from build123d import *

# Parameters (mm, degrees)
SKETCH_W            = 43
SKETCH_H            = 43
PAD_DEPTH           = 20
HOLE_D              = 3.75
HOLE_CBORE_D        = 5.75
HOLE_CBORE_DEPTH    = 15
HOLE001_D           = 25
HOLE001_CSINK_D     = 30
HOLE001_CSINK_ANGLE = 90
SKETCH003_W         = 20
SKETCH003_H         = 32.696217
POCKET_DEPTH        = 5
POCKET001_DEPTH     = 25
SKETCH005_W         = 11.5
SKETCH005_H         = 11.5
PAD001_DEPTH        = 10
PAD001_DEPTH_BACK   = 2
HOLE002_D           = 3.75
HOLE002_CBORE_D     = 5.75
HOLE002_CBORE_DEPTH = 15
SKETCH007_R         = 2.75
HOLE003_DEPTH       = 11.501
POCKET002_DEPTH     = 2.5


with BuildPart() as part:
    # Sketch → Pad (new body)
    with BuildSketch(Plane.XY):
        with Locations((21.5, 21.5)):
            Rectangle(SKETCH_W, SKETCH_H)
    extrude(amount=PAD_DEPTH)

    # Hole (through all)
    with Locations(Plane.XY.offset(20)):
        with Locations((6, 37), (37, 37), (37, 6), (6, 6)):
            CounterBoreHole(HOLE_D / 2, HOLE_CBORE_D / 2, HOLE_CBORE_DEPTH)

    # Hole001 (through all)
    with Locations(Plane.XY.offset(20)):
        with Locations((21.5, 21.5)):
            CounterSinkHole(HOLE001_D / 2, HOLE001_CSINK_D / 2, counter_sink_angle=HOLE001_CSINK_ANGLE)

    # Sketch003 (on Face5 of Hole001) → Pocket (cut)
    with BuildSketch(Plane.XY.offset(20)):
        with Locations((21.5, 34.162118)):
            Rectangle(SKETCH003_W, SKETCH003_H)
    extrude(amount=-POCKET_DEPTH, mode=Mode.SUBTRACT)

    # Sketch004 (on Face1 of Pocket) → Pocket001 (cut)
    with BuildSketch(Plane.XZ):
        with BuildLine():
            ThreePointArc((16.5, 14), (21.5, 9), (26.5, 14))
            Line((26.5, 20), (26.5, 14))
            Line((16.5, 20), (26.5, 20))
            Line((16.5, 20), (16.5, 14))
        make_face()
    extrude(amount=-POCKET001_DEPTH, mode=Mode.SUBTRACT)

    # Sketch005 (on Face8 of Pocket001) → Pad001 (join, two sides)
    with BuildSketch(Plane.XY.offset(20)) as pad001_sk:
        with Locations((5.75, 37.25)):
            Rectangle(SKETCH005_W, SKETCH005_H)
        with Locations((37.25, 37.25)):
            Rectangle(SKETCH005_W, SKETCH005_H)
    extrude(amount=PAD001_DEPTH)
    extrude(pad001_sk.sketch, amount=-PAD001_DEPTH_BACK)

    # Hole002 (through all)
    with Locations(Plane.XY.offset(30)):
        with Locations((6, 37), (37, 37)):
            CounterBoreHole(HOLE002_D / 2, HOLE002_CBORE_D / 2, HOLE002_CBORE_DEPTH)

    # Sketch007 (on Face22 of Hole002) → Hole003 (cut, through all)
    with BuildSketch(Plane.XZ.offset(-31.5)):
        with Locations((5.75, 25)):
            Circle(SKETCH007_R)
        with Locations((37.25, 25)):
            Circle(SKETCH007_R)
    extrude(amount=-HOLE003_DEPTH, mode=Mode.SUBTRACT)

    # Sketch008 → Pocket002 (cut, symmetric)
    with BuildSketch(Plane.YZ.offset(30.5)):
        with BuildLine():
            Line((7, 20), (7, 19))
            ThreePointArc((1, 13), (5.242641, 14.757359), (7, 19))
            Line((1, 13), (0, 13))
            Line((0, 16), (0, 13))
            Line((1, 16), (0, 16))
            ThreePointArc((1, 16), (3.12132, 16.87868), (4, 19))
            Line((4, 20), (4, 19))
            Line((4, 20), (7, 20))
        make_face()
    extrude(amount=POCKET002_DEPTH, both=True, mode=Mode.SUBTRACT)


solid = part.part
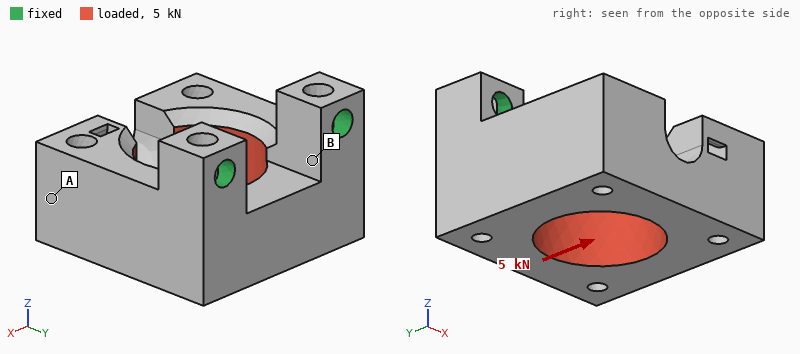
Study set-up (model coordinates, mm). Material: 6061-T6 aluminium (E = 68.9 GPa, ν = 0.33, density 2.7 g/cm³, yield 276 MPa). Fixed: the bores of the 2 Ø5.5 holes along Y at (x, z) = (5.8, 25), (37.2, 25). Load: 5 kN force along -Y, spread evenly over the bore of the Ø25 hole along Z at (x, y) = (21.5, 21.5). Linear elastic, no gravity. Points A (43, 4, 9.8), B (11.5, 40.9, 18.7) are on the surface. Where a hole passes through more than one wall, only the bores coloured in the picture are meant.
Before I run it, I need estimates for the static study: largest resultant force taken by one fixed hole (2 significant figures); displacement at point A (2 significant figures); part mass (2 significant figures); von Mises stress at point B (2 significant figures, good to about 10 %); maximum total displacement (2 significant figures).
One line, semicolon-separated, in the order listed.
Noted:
2.5 kN; 0.12 mm; 67 g; 68 MPa; 0.15 mm
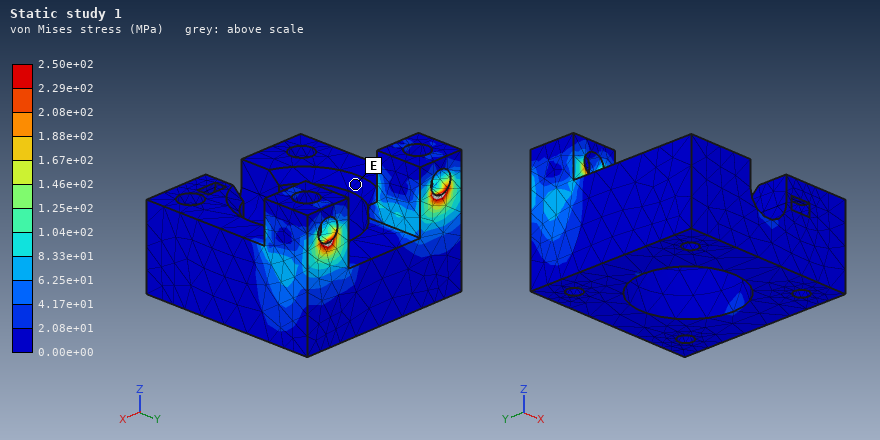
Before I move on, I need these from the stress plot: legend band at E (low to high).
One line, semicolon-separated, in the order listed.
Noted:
0.00e+00 to 2.08e+01 MPa
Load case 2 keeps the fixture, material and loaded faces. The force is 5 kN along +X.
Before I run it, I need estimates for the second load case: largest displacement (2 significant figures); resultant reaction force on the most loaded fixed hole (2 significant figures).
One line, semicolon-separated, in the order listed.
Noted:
86 µm; 3.4 kN
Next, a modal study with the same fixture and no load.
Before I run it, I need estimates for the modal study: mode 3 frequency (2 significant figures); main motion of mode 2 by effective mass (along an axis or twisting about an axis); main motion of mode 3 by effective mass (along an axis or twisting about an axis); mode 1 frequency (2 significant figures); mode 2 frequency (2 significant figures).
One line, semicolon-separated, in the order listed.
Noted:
9100 Hz; along X; along X; 3500 Hz; 5300 Hz
